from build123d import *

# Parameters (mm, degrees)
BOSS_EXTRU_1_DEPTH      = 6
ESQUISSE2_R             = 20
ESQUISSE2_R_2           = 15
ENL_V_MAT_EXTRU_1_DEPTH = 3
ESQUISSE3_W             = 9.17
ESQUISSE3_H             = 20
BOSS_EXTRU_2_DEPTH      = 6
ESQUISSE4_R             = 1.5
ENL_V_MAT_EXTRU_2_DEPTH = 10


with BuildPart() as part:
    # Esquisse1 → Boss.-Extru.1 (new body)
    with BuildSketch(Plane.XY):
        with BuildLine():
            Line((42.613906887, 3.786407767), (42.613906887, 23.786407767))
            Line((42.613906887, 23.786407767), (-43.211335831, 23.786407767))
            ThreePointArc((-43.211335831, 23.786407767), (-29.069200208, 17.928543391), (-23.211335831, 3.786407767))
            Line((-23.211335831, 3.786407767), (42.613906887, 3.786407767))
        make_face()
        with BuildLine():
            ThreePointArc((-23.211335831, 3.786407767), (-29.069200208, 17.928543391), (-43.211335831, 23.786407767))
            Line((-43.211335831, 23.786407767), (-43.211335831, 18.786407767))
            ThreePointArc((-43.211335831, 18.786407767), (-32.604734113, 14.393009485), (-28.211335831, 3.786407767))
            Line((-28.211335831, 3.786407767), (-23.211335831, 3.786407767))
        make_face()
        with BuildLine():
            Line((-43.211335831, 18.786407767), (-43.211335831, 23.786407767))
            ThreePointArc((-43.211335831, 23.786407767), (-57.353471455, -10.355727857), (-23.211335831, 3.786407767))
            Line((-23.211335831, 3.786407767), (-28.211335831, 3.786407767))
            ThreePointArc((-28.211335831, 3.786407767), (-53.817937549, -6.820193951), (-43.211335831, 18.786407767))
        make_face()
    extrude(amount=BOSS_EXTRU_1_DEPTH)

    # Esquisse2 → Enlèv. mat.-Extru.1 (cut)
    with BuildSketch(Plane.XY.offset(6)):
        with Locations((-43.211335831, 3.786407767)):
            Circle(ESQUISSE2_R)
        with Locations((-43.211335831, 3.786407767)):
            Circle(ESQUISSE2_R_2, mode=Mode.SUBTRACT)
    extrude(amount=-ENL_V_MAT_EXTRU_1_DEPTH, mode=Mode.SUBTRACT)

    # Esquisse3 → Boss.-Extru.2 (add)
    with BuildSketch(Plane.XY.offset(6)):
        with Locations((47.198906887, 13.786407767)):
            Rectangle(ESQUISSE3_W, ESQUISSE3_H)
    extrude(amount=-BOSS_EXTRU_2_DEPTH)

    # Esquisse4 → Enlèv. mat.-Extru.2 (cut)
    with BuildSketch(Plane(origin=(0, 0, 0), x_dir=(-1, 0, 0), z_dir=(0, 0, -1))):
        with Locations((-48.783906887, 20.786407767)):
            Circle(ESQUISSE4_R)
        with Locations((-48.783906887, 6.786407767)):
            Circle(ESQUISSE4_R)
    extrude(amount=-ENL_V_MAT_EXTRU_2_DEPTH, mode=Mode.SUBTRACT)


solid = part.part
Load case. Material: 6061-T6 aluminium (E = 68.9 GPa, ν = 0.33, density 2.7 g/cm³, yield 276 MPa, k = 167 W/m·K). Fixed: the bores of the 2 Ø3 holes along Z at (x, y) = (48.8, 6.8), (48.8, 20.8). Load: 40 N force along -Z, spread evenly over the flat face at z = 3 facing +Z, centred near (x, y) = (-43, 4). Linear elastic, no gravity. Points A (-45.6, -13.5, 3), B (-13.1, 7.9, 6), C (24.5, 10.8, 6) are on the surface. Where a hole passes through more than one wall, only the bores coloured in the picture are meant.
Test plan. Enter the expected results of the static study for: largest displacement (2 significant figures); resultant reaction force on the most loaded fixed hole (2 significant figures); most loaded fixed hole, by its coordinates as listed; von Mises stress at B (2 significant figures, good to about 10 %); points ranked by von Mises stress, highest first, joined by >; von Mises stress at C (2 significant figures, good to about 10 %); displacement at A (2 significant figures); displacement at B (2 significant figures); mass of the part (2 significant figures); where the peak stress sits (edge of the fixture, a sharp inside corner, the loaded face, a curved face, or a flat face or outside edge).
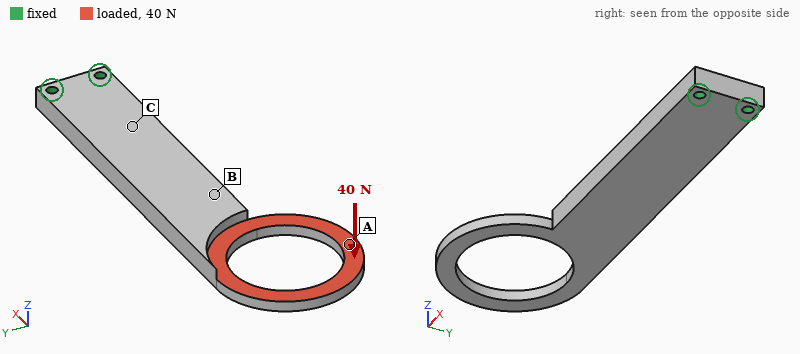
0.75 mm
45 N
(48.8, 6.8)
11 MPa
C > B > A
23 MPa
0.60 mm
0.23 mm
30 g
a curved face
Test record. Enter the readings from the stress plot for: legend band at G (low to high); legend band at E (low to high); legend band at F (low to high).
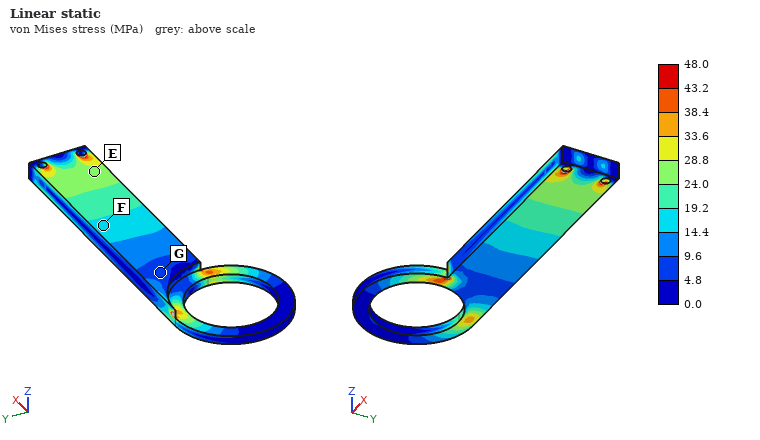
4.8 to 9.6 MPa
24.0 to 28.8 MPa
14.4 to 19.2 MPa
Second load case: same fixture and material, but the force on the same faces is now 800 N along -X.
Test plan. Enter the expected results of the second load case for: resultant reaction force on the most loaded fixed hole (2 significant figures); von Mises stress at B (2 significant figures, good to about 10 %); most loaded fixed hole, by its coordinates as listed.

940 N
17 MPa
(48.8, 6.8)
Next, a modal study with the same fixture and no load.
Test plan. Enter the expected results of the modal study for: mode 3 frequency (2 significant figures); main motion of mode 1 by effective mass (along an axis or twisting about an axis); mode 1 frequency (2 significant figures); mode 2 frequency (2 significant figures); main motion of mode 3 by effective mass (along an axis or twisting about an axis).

1700 Hz
along Z
530 Hz
1500 Hz
along Y
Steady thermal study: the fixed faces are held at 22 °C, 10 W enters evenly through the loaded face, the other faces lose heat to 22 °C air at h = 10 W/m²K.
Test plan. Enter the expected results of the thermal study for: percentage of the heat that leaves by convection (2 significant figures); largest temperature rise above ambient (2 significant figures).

14 %
71 K
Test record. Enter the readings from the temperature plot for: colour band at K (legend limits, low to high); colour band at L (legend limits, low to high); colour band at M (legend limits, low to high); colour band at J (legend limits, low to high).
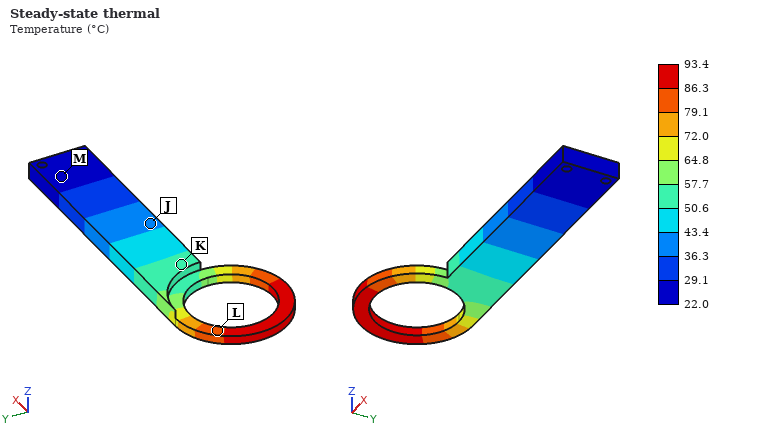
50.6 to 57.7 °C
79.1 to 86.3 °C
22.0 to 29.1 °C
36.3 to 43.4 °C
